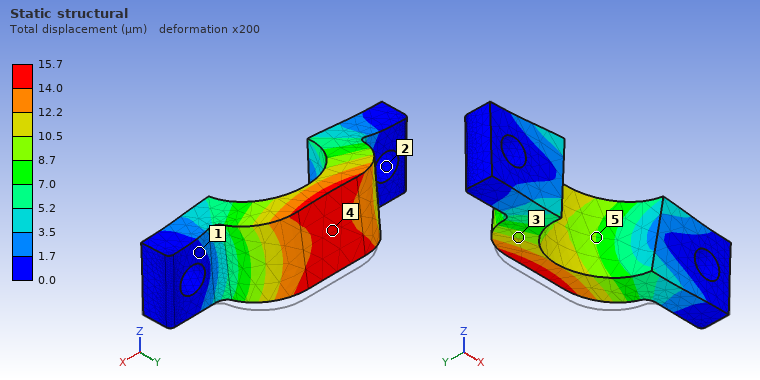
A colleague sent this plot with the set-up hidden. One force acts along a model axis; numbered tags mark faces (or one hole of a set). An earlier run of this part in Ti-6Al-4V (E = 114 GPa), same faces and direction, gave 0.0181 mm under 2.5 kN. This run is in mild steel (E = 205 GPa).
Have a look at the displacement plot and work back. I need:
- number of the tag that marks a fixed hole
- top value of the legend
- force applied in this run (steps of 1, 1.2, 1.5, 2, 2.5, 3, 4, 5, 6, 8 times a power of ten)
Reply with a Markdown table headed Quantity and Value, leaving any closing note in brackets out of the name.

| Quantity | Value |
|---|---|
| number of the tag that marks a fixed hole | 2 |
| top value of the legend | 15.7 µm |
| force applied in this run | 4 kN |
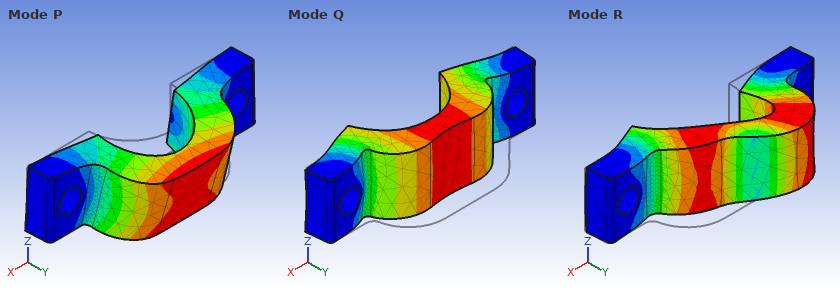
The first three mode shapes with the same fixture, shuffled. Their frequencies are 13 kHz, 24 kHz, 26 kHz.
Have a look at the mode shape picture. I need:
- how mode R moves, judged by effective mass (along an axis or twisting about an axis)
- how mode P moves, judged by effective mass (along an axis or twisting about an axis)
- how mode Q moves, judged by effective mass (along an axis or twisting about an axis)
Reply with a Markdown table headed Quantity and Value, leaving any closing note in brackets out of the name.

| Quantity | Value |
|---|---|
| how mode R moves, judged by effective mass | along X |
| how mode P moves, judged by effective mass | along Z |
| how mode Q moves, judged by effective mass | along Y |
